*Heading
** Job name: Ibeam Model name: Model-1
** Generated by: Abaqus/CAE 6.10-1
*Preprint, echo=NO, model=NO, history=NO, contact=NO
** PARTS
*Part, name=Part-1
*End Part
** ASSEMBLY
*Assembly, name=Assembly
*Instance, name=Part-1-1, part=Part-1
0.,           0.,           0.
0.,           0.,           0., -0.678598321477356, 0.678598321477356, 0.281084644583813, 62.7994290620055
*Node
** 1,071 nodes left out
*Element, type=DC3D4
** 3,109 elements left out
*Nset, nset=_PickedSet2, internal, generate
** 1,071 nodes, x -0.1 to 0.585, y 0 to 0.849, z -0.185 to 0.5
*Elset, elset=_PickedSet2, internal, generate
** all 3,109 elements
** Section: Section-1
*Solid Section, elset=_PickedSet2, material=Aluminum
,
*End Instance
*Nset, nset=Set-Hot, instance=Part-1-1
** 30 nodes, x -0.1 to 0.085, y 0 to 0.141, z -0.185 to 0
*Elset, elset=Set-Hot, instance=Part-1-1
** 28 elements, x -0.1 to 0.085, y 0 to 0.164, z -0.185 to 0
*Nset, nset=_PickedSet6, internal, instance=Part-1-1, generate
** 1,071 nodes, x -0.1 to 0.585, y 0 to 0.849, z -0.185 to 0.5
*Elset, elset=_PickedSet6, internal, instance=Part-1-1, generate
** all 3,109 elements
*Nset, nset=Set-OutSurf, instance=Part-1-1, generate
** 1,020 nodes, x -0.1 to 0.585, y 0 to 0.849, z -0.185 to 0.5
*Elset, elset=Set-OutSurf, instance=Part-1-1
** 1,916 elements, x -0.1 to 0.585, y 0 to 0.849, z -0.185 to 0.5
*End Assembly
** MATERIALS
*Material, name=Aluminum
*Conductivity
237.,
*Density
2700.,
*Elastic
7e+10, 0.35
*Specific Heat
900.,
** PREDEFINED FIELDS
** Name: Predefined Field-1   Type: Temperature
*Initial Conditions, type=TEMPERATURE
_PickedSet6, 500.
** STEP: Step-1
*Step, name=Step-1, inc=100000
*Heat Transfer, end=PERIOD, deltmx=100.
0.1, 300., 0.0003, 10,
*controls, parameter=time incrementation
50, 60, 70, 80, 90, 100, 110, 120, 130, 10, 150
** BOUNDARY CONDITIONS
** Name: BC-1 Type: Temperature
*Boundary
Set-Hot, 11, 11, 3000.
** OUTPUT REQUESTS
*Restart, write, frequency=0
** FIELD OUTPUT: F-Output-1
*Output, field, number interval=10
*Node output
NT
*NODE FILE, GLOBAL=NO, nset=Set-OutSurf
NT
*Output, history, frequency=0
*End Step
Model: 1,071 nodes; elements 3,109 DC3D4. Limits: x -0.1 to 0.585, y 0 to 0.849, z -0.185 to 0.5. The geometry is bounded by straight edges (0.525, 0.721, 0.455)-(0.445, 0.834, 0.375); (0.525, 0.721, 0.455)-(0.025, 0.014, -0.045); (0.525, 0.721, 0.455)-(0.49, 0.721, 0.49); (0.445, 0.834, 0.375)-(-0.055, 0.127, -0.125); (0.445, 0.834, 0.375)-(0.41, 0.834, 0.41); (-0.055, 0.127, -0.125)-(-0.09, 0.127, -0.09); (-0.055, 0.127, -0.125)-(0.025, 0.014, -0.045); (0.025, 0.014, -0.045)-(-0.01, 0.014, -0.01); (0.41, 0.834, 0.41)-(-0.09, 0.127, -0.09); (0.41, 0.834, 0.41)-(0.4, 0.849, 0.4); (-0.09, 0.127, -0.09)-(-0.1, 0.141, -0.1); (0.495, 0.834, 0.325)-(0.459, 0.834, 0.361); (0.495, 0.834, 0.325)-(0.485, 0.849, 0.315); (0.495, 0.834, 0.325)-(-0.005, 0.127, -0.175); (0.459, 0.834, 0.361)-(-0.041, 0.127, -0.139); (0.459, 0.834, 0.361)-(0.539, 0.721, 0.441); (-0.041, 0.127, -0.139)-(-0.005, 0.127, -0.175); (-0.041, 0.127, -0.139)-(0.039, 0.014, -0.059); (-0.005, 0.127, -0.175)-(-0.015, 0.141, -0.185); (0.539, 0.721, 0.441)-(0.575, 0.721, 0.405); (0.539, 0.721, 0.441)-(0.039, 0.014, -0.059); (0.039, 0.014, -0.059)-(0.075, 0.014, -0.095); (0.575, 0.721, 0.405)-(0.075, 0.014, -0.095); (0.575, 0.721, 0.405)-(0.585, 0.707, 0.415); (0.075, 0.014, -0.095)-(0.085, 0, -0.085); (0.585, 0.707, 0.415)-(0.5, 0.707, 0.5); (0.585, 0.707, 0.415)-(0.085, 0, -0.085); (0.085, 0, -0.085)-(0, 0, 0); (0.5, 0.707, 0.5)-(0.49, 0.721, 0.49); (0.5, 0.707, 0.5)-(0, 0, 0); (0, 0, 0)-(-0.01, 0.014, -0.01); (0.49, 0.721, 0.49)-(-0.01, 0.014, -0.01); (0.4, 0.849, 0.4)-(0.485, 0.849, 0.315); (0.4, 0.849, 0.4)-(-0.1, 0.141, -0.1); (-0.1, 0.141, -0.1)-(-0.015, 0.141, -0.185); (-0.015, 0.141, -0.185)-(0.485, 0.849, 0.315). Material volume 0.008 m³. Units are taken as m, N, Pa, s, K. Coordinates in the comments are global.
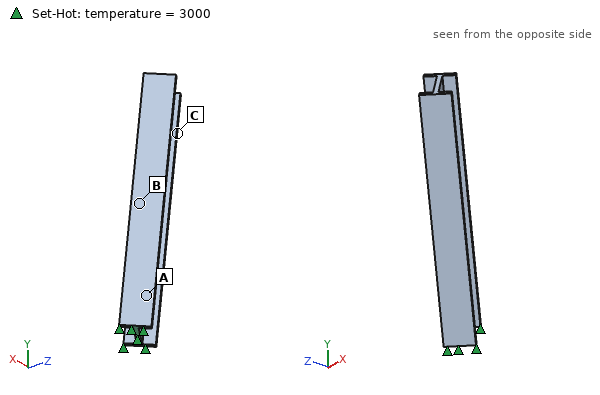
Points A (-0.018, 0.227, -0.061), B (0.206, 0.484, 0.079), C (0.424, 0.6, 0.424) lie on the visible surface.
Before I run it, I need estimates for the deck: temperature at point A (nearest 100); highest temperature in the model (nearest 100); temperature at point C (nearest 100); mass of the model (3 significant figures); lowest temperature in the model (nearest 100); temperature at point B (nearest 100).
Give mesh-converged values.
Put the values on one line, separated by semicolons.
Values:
2000 K; 3000 K; 500 K; 21.6 kg; 500 K; 600 K
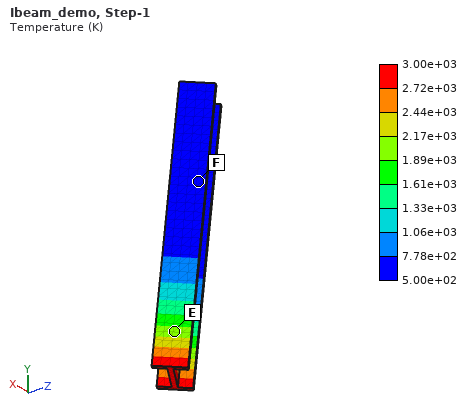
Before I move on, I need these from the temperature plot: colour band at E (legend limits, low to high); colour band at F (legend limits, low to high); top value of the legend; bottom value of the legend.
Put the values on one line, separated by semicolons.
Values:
1.89e+03 to 2.17e+03 K; 5.00e+02 to 7.78e+02 K; 3.00e+03 K; 5.00e+02 K
